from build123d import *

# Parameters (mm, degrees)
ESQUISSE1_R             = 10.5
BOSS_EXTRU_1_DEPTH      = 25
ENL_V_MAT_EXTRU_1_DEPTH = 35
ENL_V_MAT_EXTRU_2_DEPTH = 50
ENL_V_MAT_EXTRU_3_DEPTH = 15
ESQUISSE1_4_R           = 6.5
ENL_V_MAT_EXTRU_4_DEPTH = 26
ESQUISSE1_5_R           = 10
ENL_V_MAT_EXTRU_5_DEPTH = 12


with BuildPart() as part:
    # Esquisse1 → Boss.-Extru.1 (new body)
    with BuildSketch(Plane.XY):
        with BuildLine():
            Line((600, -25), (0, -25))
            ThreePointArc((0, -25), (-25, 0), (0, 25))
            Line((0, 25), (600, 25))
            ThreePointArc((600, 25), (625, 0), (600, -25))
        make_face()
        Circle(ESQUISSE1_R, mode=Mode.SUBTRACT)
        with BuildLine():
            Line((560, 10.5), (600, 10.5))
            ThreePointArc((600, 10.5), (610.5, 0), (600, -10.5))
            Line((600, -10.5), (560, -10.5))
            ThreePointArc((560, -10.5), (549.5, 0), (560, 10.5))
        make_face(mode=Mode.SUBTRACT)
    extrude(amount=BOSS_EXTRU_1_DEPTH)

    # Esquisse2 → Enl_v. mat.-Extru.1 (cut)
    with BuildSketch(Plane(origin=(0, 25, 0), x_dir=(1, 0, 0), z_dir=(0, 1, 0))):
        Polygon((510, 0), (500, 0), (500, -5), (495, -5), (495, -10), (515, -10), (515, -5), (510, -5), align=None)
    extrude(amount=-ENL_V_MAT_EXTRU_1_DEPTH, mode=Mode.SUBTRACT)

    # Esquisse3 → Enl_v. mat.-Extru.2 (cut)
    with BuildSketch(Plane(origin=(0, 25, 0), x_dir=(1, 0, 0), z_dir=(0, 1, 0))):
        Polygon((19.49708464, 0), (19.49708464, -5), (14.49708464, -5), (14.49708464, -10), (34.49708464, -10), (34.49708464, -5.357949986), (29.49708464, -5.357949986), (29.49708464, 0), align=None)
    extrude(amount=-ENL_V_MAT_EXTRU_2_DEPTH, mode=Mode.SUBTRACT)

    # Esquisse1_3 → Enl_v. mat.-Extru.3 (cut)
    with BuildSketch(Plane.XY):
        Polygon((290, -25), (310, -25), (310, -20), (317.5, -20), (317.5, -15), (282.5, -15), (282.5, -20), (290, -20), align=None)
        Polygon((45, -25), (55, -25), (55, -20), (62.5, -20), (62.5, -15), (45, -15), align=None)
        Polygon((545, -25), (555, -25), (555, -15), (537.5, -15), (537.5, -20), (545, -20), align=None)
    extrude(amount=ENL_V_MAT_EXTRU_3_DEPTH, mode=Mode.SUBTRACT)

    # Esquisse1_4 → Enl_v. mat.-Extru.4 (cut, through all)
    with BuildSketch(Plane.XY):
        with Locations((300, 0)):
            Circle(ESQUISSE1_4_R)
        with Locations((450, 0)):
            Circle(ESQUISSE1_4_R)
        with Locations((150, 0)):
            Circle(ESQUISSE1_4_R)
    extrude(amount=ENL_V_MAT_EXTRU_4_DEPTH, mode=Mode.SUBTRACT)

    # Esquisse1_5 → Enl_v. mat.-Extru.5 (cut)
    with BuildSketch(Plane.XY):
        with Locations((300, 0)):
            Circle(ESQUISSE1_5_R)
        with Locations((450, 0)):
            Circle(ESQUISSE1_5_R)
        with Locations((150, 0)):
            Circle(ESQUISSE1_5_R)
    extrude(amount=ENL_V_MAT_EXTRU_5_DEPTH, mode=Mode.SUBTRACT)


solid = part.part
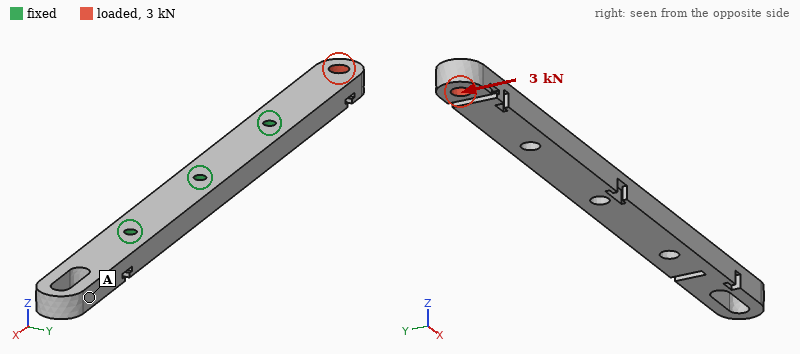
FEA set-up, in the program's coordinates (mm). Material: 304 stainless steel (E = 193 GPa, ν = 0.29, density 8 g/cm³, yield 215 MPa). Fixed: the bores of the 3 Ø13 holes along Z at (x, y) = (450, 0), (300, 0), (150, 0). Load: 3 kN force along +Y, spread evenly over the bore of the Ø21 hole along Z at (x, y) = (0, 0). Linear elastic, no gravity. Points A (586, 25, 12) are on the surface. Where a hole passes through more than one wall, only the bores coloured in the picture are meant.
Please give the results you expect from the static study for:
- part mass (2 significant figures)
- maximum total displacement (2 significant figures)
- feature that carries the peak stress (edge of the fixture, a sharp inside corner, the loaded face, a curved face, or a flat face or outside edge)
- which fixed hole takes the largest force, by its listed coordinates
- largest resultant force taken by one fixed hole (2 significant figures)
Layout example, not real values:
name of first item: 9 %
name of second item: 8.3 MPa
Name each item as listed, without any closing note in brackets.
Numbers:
part mass: 5.8 kg
maximum total displacement: 0.15 mm
feature that carries the peak stress: edge of the fixture
which fixed hole takes the largest force, by its listed coordinates: (150, 0)
largest resultant force taken by one fixed hole: 5.2 kN
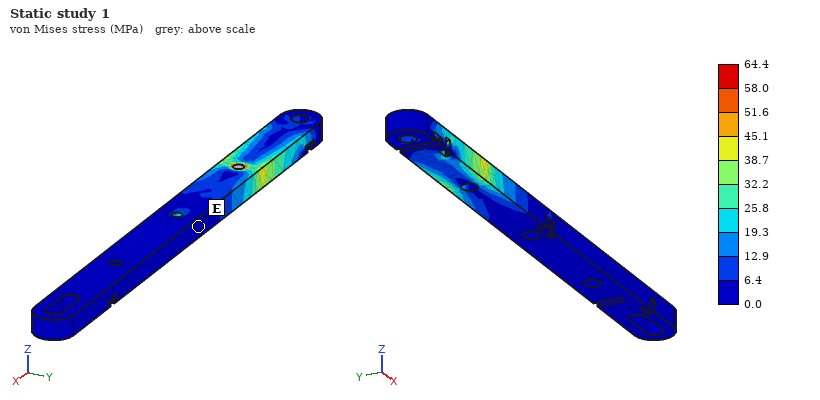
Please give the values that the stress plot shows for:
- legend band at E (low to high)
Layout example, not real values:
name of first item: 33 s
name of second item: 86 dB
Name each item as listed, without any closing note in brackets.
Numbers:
legend band at E: 0.0 to 6.4 MPa
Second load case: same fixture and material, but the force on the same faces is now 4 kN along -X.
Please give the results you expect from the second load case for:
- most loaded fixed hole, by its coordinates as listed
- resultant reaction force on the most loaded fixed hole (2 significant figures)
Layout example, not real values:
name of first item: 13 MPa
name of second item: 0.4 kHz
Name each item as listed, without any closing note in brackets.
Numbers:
most loaded fixed hole, by its coordinates as listed: (150, 0)
resultant reaction force on the most loaded fixed hole: 3.4 kN
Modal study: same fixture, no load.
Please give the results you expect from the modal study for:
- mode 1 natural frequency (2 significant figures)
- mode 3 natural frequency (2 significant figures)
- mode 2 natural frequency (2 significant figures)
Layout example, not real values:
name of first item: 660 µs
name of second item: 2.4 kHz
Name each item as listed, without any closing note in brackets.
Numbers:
mode 1 natural frequency: 600 Hz
mode 3 natural frequency: 1100 Hz
mode 2 natural frequency: 620 Hz
